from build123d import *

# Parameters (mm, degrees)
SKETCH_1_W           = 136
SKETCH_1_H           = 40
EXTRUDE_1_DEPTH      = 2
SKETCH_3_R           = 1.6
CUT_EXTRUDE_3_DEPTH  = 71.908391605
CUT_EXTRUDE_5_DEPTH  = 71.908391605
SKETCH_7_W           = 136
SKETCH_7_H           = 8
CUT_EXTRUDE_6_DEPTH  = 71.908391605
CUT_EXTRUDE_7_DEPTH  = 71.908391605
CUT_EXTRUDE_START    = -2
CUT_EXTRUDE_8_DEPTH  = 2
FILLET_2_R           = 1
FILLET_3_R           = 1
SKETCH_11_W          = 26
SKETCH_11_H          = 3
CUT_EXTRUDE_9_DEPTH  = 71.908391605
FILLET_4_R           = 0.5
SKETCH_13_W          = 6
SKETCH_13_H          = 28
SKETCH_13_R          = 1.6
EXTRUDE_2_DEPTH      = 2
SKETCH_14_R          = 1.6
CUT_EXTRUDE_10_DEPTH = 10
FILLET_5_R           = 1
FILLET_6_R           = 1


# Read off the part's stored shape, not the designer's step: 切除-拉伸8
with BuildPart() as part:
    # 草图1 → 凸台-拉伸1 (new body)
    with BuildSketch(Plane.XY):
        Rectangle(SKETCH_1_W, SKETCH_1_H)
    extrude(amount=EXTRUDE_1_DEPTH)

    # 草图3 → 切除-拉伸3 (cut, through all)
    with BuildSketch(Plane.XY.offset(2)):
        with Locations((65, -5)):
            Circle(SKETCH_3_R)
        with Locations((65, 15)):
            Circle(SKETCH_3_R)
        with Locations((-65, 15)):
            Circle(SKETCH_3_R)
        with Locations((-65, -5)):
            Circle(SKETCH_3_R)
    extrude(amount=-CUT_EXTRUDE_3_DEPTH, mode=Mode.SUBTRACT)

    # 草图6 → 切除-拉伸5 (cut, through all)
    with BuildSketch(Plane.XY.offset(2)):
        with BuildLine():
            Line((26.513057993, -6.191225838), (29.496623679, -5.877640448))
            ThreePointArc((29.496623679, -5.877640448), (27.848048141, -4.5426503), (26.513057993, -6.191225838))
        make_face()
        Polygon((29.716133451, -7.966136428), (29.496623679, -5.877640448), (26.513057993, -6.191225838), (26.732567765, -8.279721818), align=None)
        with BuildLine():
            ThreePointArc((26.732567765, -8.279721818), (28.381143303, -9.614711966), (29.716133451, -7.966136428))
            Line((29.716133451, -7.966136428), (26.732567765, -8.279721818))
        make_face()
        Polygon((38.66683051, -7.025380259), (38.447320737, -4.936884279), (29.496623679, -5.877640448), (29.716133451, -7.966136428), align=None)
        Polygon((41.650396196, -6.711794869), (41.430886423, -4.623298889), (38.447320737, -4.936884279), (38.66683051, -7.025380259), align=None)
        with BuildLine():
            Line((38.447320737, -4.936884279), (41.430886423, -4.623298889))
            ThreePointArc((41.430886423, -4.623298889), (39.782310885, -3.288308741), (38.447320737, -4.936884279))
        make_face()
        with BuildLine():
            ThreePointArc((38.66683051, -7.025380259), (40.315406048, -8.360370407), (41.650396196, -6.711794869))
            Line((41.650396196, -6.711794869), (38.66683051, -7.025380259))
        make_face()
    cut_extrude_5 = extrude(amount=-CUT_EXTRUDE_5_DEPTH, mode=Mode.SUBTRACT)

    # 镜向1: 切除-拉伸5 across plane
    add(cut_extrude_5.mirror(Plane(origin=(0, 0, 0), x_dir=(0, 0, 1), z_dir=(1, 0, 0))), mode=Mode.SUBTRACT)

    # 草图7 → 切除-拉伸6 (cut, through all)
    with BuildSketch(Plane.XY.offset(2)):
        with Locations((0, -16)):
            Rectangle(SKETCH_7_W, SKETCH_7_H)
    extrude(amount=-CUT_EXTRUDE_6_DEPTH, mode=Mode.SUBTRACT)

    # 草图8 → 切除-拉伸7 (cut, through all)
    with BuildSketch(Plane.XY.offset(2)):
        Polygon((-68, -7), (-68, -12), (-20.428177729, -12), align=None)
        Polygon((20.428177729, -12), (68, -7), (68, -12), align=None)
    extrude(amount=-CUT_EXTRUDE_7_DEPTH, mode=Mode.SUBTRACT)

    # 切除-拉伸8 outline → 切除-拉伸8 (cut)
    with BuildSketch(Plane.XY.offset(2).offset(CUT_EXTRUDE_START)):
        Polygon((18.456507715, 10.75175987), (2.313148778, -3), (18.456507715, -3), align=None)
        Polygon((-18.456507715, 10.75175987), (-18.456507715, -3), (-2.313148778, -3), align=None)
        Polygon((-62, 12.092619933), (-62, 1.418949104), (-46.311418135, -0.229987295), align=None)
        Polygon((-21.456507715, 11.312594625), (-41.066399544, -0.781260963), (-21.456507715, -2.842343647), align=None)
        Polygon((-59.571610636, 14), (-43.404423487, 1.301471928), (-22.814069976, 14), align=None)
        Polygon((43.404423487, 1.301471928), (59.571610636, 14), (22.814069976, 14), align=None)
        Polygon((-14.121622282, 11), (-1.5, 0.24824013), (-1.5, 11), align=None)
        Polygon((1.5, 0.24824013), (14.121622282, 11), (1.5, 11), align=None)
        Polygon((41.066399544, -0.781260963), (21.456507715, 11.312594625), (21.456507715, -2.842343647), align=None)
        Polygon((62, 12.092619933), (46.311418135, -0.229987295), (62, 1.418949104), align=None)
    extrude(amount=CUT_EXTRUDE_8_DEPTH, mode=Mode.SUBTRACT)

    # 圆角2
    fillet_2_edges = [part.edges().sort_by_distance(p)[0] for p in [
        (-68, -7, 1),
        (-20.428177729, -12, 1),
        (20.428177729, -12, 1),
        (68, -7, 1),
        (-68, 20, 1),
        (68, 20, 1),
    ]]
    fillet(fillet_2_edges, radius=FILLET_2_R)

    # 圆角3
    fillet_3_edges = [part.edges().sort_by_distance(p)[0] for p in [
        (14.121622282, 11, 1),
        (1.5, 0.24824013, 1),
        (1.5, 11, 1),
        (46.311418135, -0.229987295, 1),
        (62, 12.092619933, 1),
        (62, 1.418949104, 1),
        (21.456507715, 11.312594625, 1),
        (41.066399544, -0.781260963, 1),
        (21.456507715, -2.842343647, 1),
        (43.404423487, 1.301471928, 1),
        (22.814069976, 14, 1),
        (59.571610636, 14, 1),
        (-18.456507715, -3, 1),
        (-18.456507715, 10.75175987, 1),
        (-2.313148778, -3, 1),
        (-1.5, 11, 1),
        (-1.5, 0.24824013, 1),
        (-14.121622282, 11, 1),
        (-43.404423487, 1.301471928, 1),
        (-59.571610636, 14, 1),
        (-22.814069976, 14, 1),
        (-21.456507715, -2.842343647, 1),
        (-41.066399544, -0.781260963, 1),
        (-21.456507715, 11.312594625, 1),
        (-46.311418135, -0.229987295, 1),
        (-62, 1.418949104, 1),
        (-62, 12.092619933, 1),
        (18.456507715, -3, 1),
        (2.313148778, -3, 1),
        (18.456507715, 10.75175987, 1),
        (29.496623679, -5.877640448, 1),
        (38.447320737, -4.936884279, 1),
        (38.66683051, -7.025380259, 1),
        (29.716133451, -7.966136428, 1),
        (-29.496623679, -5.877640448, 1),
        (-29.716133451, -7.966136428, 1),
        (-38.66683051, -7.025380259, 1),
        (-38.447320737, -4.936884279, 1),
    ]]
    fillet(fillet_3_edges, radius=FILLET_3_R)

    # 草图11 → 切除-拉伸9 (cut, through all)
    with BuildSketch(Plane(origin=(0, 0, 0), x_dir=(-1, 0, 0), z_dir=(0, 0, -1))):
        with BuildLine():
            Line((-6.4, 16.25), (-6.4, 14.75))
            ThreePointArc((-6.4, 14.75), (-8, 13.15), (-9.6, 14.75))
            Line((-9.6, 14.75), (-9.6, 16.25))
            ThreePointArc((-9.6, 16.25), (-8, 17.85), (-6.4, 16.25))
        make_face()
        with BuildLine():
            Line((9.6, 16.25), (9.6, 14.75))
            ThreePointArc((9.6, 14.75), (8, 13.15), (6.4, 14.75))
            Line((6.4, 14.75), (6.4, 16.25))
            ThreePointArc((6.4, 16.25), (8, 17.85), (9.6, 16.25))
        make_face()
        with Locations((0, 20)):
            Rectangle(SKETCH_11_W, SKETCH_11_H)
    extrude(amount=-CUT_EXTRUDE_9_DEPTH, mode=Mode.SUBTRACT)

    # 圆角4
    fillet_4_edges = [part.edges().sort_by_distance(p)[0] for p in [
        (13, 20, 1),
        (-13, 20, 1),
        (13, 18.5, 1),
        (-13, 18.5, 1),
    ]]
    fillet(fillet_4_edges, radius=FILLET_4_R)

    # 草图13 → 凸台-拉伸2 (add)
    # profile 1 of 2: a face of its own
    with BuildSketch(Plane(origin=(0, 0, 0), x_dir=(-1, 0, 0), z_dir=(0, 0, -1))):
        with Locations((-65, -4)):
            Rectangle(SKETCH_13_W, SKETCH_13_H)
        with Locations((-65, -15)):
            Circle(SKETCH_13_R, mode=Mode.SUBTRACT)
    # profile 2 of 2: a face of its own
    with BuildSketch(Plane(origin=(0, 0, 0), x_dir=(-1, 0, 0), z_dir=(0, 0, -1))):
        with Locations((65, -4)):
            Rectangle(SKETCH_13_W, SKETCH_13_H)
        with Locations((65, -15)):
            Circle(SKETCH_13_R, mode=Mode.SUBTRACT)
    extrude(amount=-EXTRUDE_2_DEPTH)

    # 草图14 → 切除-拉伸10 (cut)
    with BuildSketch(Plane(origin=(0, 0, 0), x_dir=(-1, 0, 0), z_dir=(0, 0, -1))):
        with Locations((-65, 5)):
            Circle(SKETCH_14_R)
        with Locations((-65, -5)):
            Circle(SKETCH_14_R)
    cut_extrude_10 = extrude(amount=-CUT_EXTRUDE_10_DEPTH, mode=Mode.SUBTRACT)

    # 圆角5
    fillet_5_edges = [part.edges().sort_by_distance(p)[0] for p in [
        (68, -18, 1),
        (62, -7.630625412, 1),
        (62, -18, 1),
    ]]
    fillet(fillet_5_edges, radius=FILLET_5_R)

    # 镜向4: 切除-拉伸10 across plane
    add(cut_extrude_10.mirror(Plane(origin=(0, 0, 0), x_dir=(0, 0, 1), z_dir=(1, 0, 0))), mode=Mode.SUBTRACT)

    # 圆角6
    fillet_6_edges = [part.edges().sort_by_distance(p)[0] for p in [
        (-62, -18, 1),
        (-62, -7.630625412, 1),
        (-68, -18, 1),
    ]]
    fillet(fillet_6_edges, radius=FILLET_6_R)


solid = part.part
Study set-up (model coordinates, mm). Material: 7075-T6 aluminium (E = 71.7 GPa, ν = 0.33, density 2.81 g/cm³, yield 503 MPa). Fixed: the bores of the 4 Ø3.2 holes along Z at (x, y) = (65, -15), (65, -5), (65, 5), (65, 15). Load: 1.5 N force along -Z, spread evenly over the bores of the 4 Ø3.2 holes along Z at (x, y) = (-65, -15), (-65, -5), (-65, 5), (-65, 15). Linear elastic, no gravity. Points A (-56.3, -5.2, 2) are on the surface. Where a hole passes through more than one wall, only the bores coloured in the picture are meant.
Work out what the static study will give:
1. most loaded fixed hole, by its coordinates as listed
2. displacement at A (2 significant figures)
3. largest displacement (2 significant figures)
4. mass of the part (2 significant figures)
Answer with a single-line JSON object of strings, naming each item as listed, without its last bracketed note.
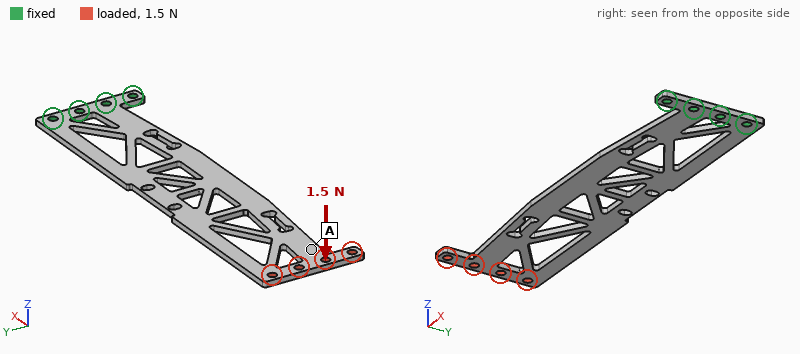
{"most loaded fixed hole, by its coordinates as listed": "(65, -5)", "displacement at A": "1.2 mm", "largest displacement": "1.4 mm", "mass of the part": "16 g"}
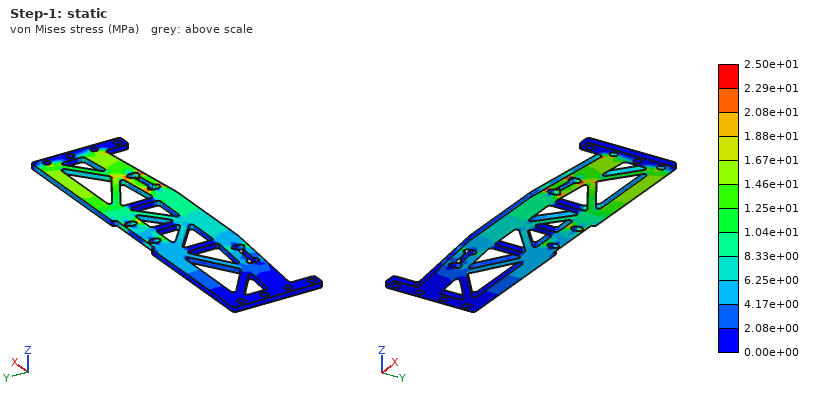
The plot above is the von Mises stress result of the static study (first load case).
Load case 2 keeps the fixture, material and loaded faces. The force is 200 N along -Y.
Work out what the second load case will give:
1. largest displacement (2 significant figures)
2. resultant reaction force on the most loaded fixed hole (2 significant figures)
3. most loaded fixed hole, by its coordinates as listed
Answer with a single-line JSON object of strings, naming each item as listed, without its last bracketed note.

{"largest displacement": "0.83 mm", "resultant reaction force on the most loaded fixed hole": "1.2 kN", "most loaded fixed hole, by its coordinates as listed": "(65, 15)"}
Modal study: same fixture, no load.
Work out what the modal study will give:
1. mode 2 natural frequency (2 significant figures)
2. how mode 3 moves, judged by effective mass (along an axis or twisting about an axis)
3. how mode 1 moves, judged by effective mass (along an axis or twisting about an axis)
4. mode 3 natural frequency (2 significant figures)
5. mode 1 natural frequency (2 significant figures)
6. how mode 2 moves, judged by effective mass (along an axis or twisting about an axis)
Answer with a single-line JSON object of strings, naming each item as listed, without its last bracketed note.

{"mode 2 natural frequency": "510 Hz", "how mode 3 moves, judged by effective mass": "twisting about X", "how mode 1 moves, judged by effective mass": "along Z", "mode 3 natural frequency": "590 Hz", "mode 1 natural frequency": "83 Hz", "how mode 2 moves, judged by effective mass": "along Z"}
